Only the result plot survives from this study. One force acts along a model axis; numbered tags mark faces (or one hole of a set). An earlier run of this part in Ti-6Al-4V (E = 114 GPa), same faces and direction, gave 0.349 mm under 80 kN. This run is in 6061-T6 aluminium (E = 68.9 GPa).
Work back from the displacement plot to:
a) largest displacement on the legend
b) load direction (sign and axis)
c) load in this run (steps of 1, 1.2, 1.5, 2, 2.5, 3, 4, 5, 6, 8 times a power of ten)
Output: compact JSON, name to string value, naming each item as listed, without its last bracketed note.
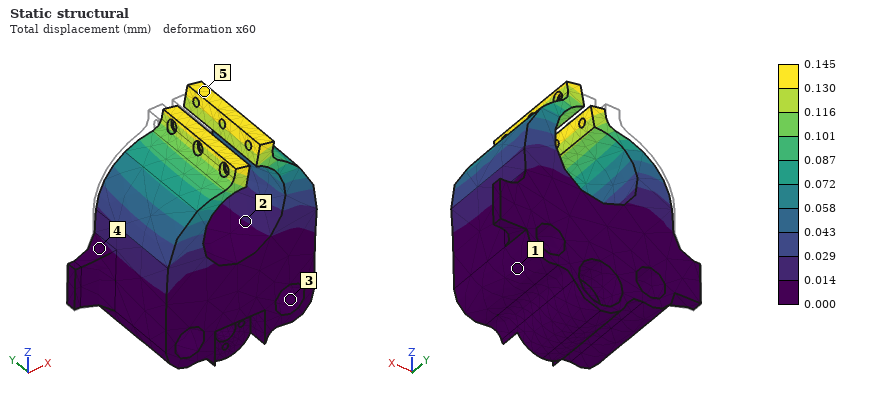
{"largest displacement on the legend": "0.145 mm", "load direction": "+X", "load in this run": "20 kN"}
